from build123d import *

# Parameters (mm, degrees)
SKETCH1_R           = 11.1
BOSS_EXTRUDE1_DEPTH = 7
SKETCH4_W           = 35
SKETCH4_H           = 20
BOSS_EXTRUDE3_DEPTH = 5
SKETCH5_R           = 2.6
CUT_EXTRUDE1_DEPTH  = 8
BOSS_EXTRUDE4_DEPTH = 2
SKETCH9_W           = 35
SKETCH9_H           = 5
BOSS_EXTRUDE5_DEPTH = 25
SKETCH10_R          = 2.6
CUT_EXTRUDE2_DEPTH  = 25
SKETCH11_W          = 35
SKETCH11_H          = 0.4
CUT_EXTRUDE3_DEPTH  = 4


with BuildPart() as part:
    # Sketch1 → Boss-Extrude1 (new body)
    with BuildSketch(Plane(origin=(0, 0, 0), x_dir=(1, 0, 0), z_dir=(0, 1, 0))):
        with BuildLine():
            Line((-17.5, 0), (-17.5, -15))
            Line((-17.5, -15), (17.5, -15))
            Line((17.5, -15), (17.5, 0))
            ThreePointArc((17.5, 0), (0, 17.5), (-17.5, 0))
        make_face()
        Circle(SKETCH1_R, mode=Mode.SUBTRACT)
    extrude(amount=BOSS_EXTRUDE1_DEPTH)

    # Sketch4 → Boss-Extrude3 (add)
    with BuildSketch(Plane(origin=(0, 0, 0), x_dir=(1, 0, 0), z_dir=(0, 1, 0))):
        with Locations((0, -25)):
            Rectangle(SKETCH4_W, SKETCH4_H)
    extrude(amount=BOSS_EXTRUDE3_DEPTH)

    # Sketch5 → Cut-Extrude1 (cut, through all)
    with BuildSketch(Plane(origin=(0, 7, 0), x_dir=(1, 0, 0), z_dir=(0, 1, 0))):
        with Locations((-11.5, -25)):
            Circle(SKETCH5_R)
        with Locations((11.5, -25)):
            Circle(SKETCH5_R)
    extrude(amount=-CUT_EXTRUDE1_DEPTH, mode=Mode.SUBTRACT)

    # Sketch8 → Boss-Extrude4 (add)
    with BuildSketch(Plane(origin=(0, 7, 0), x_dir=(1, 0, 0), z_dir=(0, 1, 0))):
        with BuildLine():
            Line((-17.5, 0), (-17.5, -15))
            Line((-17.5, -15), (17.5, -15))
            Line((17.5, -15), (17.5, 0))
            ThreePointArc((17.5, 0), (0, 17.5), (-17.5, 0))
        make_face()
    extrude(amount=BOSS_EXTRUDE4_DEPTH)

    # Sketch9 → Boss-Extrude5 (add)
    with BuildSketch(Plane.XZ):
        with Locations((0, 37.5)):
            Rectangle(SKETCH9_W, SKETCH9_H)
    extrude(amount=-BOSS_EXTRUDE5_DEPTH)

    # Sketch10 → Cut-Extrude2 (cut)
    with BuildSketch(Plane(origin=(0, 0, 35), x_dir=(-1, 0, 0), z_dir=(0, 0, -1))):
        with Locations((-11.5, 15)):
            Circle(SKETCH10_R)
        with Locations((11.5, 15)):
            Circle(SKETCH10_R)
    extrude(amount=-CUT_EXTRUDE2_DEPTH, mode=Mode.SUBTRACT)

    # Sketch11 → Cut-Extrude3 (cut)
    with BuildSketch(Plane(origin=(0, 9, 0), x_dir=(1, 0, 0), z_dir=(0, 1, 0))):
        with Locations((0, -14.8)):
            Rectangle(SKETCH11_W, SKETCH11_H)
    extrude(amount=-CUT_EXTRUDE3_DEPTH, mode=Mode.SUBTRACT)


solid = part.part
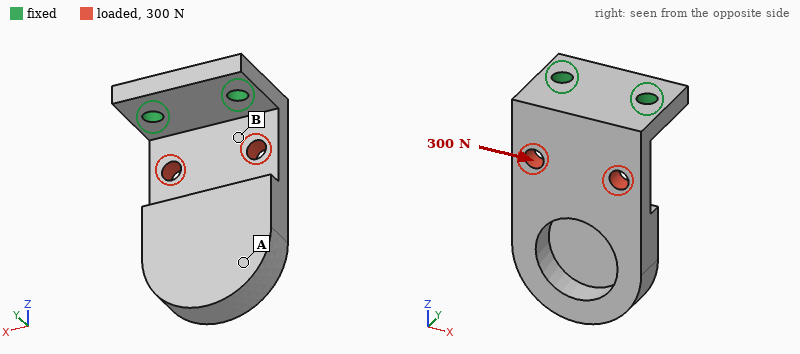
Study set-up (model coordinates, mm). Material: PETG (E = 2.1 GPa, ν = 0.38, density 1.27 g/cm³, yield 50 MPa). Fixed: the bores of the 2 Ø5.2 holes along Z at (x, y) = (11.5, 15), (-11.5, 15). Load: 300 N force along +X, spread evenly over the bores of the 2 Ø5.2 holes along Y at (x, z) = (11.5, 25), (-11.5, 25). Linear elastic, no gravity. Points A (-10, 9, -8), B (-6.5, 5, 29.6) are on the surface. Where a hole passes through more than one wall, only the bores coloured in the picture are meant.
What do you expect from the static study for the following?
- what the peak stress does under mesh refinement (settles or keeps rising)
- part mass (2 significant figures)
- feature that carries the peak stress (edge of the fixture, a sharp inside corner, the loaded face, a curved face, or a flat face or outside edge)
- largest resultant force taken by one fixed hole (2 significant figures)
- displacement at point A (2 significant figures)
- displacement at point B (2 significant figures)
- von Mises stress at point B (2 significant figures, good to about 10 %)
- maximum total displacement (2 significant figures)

keeps rising
17 g
edge of the fixture
250 N
0.61 mm
0.15 mm
6.8 MPa
0.70 mm
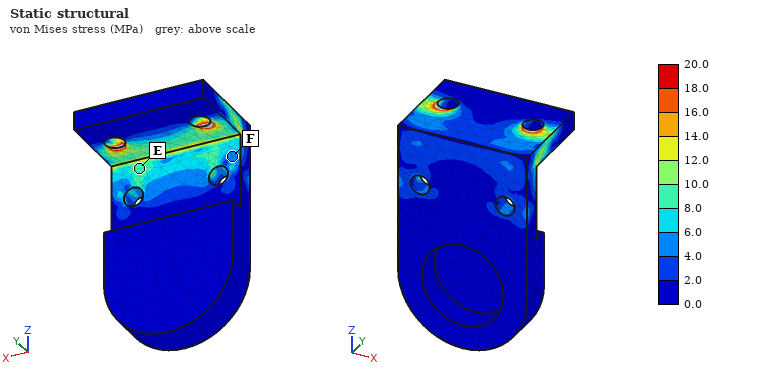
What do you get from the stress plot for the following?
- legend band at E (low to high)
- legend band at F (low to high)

8.0 to 10.0 MPa
4.0 to 6.0 MPa
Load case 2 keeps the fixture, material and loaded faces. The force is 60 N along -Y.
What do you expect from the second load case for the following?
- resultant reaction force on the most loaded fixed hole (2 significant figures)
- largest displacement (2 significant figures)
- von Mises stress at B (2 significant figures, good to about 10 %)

31 N
0.79 mm
1.9 MPa
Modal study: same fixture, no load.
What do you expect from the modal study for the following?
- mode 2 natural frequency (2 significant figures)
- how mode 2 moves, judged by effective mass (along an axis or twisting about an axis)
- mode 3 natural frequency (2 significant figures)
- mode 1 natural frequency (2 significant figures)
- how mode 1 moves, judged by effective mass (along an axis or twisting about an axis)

680 Hz
along X
1200 Hz
260 Hz
along Y
